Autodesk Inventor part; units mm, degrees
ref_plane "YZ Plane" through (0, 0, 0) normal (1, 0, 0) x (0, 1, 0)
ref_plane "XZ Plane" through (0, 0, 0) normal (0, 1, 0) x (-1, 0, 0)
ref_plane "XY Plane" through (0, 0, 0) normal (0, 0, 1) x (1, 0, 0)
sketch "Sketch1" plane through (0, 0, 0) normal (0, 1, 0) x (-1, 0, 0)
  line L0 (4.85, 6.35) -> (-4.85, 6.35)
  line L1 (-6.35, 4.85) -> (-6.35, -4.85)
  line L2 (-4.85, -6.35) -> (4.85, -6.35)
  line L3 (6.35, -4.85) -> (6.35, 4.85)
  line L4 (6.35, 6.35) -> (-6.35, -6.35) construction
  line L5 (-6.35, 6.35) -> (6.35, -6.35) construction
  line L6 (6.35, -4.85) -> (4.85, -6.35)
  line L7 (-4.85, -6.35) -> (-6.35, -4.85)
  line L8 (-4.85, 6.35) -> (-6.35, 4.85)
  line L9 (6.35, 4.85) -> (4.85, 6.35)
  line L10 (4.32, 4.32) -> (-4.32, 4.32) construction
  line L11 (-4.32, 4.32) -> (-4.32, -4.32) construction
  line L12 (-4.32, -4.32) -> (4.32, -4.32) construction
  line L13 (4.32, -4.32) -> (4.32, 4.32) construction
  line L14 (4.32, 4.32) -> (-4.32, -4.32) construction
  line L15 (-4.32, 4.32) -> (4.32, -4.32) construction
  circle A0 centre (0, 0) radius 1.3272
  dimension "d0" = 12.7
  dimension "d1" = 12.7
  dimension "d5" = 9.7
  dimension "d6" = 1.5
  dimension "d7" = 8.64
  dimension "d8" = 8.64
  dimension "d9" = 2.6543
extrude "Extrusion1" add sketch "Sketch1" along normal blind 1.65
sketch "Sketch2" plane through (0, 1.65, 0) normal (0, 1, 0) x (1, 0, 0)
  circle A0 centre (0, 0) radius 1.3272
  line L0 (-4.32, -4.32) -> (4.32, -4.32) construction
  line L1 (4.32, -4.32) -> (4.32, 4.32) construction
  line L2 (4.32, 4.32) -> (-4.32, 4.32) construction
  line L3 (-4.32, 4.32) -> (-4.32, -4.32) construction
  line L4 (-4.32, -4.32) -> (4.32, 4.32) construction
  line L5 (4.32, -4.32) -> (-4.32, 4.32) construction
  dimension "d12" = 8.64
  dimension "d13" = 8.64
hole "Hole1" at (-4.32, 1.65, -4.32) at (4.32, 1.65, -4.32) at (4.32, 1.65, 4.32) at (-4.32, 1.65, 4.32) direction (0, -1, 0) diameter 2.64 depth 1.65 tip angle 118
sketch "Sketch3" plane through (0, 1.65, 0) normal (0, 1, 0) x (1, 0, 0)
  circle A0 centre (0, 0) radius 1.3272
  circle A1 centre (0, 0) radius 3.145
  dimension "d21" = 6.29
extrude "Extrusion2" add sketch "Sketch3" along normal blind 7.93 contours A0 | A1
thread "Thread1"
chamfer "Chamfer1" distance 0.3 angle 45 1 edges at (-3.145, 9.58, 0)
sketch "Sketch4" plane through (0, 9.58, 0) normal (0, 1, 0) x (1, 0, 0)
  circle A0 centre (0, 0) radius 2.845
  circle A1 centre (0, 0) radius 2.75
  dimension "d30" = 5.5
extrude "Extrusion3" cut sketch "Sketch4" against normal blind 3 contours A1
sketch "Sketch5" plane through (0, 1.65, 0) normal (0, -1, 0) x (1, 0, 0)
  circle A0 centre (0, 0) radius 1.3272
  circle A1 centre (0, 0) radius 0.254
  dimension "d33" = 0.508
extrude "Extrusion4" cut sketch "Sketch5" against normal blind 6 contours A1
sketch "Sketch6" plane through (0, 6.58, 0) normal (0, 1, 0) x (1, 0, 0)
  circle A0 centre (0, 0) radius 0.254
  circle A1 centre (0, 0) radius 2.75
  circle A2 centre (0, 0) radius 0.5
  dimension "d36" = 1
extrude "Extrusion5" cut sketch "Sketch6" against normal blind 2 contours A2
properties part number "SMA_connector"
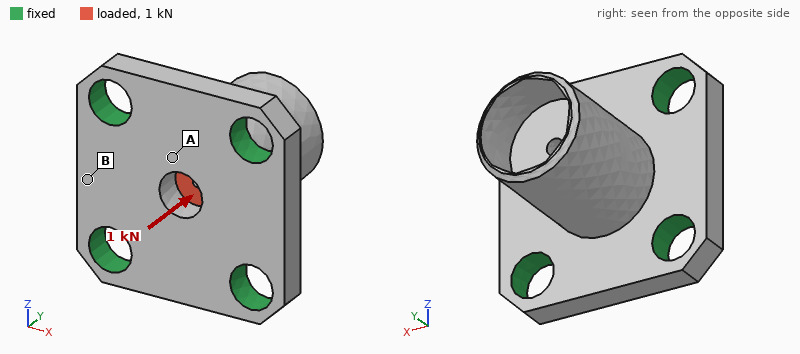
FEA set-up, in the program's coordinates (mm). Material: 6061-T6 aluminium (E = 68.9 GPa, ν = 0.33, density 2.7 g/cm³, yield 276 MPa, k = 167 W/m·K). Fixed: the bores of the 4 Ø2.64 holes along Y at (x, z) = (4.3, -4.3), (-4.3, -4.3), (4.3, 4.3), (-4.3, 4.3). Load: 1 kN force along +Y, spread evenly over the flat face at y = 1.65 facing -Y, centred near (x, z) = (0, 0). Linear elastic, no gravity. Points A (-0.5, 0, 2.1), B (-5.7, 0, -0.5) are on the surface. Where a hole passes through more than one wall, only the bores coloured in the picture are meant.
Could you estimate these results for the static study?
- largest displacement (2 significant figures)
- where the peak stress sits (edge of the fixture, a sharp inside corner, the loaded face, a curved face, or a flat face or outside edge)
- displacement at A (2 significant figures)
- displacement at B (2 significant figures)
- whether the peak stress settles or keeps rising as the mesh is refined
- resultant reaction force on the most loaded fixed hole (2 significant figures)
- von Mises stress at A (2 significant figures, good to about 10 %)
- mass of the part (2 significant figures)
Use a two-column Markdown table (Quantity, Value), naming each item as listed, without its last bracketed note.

| Quantity | Value |
|---|---|
| largest displacement | 13 µm |
| where the peak stress sits | edge of the fixture |
| displacement at A | 8.2 µm |
| displacement at B | 2.1 µm |
| whether the peak stress settles or keeps rising as the mesh is refined | keeps rising |
| resultant reaction force on the most loaded fixed hole | 280 N |
| von Mises stress at A | 66 MPa |
| mass of the part | 1.0 g |
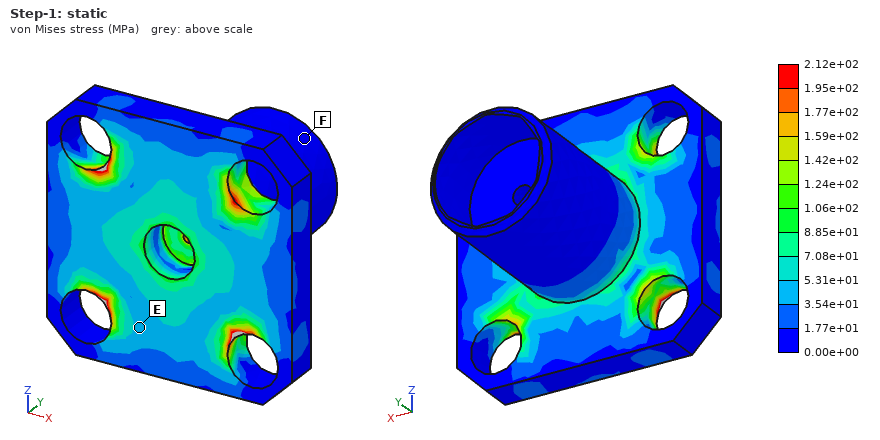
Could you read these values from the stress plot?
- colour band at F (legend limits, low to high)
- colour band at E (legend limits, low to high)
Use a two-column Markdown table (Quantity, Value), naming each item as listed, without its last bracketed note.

| Quantity | Value |
|---|---|
| colour band at F | 0.00e+00 to 1.77e+01 MPa |
| colour band at E | 3.54e+01 to 5.31e+01 MPa |
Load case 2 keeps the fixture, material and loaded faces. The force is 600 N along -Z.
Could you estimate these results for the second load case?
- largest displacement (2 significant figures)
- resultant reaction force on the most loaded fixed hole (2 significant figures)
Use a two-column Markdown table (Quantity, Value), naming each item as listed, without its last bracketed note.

| Quantity | Value |
|---|---|
| largest displacement | 5.8 µm |
| resultant reaction force on the most loaded fixed hole | 170 N |
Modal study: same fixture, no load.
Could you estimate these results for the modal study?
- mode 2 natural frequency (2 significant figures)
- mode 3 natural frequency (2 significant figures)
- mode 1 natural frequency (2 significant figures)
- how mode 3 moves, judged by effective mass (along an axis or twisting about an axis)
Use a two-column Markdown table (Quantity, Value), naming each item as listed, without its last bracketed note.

| Quantity | Value |
|---|---|
| mode 2 natural frequency | 47 kHz |
| mode 3 natural frequency | 71 kHz |
| mode 1 natural frequency | 47 kHz |
| how mode 3 moves, judged by effective mass | along Y |
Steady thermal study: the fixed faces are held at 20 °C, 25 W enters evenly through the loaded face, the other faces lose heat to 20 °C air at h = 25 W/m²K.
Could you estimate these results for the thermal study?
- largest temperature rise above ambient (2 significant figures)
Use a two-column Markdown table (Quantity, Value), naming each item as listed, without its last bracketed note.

| Quantity | Value |
|---|---|
| largest temperature rise above ambient | 40 K |
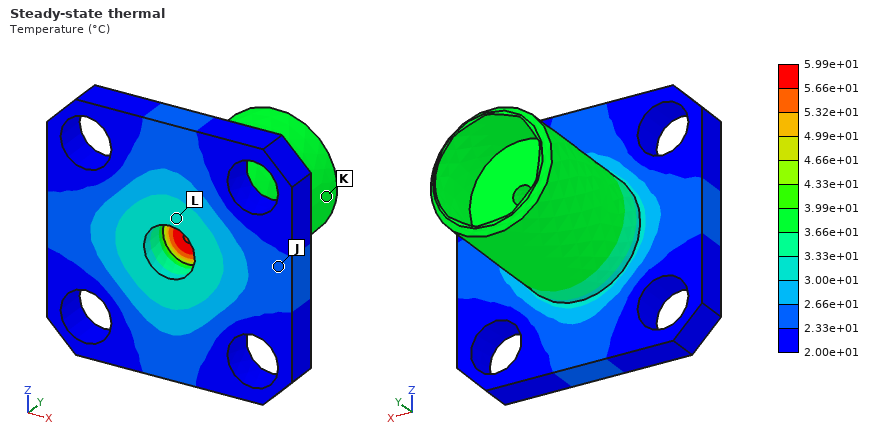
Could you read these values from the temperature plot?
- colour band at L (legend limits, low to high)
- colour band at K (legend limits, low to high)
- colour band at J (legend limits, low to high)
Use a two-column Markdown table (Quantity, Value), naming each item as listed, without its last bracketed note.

| Quantity | Value |
|---|---|
| colour band at L | 3.00e+01 to 3.33e+01 °C |
| colour band at K | 3.66e+01 to 3.99e+01 °C |
| colour band at J | 2.33e+01 to 2.66e+01 °C |
